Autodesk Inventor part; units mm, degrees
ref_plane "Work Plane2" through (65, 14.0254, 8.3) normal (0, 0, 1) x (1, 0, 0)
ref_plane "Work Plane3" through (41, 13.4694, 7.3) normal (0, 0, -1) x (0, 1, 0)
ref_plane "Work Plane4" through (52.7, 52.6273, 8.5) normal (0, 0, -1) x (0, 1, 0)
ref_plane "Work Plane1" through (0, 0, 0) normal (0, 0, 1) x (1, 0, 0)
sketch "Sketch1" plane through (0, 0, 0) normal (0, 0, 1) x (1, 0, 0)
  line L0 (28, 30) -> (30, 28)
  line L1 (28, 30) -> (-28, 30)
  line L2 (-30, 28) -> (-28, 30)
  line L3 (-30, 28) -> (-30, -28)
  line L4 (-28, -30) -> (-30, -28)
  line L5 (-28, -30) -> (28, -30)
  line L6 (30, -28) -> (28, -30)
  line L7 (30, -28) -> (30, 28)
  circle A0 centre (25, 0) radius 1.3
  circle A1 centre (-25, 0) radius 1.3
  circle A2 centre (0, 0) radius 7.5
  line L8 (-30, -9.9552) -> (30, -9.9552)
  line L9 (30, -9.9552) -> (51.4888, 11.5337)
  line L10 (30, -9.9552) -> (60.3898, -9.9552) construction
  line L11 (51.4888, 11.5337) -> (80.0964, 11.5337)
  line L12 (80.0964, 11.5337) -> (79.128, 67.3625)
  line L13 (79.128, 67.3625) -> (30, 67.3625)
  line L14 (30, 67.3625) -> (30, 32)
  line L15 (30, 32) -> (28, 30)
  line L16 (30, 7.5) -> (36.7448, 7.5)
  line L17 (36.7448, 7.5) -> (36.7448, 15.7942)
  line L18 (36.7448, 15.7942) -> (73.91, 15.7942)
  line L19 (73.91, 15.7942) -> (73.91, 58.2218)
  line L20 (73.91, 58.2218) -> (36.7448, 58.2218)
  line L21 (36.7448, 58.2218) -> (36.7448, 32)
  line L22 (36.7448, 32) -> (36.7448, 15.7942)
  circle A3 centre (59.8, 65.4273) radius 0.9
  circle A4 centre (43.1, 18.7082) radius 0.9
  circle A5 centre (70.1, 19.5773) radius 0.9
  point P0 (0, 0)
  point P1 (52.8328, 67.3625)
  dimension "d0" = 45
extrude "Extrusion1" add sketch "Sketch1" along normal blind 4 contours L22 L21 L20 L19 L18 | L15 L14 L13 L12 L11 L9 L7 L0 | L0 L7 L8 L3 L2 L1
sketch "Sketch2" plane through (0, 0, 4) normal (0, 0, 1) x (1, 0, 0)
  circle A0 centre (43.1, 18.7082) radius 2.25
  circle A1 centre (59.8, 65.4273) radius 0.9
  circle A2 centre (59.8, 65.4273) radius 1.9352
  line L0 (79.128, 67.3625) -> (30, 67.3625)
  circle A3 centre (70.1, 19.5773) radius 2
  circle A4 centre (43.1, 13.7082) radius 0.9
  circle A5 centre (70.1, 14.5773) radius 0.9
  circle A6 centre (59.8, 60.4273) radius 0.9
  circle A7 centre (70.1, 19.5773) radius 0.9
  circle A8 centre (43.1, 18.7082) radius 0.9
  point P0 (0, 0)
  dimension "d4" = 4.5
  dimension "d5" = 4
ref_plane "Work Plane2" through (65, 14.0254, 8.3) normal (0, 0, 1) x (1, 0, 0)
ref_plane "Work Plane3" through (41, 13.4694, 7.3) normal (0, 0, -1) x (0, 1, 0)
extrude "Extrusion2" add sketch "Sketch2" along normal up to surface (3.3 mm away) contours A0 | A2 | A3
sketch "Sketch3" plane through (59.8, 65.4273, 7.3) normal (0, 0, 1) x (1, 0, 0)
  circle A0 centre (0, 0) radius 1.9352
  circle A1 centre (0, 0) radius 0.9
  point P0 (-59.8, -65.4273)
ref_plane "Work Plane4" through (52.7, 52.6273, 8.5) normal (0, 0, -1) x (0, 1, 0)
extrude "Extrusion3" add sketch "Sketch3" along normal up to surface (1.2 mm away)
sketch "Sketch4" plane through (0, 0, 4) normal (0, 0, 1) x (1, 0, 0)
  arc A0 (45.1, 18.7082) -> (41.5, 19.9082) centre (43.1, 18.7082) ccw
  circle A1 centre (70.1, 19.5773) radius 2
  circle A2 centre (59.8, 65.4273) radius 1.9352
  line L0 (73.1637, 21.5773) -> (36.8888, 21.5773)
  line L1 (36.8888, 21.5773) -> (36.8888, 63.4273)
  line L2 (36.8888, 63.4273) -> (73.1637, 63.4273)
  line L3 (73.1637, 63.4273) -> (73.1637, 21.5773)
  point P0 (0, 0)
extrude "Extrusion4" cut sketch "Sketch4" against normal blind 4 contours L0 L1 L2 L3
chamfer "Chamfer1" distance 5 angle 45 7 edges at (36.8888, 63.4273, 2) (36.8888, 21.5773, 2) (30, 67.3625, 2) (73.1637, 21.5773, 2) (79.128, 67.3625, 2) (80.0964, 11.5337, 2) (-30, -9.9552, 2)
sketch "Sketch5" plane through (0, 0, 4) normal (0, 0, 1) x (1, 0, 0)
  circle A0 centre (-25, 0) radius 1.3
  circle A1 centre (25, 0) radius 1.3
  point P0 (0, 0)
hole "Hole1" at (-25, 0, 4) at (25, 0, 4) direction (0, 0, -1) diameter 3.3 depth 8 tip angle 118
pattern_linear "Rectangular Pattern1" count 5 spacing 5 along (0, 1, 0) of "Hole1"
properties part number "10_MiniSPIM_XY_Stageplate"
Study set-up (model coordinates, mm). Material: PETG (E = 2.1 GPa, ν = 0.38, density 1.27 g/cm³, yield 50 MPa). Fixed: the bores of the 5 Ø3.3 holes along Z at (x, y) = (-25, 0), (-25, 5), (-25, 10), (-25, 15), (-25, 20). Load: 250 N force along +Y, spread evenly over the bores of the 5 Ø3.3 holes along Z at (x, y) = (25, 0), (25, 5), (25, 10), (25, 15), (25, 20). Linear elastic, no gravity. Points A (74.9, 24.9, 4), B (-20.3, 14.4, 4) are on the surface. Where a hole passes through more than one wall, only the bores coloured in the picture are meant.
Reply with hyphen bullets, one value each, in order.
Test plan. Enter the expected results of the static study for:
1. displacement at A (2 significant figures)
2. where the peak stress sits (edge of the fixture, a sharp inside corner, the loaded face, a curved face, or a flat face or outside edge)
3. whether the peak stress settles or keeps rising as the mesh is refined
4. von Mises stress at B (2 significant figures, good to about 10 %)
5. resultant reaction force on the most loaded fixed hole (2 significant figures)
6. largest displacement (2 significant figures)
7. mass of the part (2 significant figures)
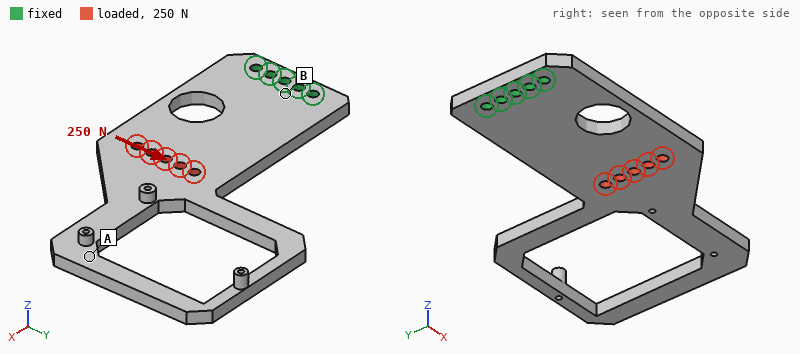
- 1.3 mm
- edge of the fixture
- keeps rising
- 8.3 MPa
- 530 N
- 1.5 mm
- 18 g
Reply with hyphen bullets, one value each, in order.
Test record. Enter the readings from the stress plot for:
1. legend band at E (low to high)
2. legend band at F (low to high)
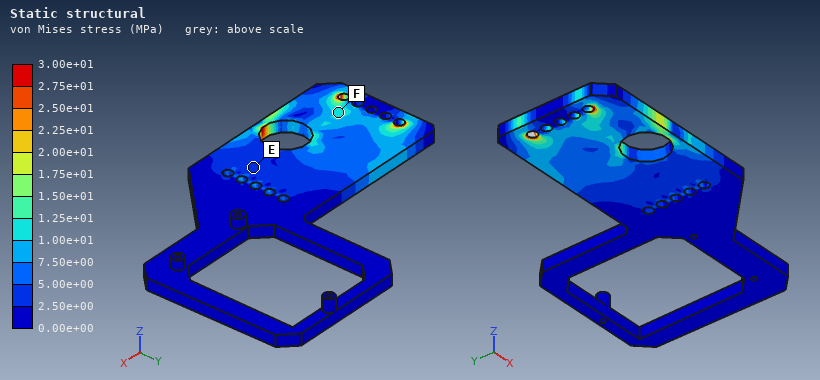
- 2.50e+00 to 5.00e+00 MPa
- 1.00e+01 to 1.25e+01 MPa
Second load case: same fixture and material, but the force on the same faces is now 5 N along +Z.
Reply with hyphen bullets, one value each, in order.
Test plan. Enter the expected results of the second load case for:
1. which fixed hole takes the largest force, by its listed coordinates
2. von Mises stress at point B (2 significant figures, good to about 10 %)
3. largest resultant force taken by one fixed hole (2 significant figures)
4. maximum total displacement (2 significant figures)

- (-25, 15)
- 2.3 MPa
- 2.7 N
- 1.4 mm
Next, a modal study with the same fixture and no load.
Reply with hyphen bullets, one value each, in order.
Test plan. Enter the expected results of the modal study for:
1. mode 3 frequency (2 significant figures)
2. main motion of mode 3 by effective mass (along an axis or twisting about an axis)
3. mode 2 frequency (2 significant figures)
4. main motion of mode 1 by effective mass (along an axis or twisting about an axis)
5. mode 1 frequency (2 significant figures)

- 350 Hz
- along Z
- 210 Hz
- along Z
- 78 Hz
